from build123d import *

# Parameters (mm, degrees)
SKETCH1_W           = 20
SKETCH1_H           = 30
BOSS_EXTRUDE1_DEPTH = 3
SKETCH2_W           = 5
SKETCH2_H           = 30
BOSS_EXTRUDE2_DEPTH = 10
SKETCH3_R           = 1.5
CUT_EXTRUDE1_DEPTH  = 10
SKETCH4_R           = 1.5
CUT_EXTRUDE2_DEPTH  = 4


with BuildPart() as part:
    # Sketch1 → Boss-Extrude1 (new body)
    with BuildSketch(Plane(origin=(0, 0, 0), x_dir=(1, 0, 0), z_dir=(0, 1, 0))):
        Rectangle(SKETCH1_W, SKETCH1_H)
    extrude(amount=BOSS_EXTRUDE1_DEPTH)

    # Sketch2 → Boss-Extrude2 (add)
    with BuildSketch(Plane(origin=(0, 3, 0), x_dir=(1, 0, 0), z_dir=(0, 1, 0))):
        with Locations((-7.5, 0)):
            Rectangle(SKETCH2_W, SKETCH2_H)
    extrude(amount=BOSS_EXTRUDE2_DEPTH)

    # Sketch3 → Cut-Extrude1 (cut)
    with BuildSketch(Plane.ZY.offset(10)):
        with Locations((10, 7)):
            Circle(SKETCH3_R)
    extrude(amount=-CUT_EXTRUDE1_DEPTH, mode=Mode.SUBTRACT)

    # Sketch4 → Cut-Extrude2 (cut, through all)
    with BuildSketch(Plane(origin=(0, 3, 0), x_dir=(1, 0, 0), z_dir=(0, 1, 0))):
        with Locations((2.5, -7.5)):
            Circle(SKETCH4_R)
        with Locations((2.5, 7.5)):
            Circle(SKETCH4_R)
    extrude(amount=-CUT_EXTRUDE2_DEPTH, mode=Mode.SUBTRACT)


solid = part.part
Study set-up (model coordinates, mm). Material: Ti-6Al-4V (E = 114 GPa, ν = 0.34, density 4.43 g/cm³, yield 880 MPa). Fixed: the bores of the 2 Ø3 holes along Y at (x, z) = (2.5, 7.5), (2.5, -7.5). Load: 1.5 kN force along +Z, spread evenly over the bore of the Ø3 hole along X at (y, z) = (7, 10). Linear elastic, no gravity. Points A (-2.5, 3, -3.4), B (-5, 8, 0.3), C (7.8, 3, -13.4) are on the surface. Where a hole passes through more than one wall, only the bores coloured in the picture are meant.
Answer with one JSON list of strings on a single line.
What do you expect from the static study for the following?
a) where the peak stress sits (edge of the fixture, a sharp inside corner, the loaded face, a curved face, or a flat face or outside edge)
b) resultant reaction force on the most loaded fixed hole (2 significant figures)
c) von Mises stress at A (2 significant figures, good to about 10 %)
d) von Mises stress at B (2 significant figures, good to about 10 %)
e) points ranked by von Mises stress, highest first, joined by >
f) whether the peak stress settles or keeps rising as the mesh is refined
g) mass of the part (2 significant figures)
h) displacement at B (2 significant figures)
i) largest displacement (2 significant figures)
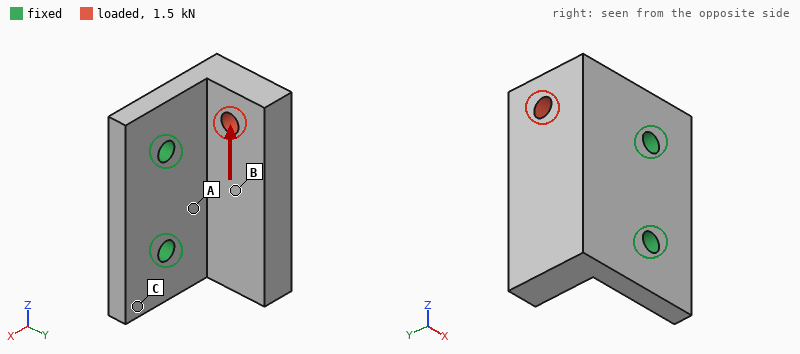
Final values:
["edge of the fixture", "1.2 kN", "85 MPa", "35 MPa", "A > B > C", "keeps rising", "14 g", "17 µm", "36 µm"]
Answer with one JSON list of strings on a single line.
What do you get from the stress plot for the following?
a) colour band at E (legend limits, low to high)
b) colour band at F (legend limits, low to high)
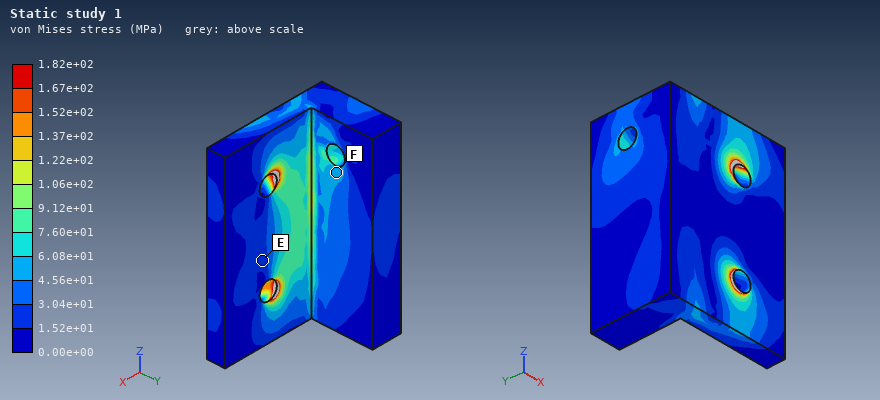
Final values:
["1.52e+01 to 3.04e+01 MPa", "4.56e+01 to 6.08e+01 MPa"]
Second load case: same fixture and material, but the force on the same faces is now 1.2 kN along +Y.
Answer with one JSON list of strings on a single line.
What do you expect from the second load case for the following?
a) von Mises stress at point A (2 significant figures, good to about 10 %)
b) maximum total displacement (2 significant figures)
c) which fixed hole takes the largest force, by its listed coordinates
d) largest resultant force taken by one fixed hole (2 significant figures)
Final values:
["120 MPa", "0.16 mm", "(2.5, 7.5)", "1.2 kN"]
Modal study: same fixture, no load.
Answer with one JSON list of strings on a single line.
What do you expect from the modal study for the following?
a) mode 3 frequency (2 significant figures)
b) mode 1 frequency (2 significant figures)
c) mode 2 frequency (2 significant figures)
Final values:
["20 kHz", "5800 Hz", "11 kHz"]
